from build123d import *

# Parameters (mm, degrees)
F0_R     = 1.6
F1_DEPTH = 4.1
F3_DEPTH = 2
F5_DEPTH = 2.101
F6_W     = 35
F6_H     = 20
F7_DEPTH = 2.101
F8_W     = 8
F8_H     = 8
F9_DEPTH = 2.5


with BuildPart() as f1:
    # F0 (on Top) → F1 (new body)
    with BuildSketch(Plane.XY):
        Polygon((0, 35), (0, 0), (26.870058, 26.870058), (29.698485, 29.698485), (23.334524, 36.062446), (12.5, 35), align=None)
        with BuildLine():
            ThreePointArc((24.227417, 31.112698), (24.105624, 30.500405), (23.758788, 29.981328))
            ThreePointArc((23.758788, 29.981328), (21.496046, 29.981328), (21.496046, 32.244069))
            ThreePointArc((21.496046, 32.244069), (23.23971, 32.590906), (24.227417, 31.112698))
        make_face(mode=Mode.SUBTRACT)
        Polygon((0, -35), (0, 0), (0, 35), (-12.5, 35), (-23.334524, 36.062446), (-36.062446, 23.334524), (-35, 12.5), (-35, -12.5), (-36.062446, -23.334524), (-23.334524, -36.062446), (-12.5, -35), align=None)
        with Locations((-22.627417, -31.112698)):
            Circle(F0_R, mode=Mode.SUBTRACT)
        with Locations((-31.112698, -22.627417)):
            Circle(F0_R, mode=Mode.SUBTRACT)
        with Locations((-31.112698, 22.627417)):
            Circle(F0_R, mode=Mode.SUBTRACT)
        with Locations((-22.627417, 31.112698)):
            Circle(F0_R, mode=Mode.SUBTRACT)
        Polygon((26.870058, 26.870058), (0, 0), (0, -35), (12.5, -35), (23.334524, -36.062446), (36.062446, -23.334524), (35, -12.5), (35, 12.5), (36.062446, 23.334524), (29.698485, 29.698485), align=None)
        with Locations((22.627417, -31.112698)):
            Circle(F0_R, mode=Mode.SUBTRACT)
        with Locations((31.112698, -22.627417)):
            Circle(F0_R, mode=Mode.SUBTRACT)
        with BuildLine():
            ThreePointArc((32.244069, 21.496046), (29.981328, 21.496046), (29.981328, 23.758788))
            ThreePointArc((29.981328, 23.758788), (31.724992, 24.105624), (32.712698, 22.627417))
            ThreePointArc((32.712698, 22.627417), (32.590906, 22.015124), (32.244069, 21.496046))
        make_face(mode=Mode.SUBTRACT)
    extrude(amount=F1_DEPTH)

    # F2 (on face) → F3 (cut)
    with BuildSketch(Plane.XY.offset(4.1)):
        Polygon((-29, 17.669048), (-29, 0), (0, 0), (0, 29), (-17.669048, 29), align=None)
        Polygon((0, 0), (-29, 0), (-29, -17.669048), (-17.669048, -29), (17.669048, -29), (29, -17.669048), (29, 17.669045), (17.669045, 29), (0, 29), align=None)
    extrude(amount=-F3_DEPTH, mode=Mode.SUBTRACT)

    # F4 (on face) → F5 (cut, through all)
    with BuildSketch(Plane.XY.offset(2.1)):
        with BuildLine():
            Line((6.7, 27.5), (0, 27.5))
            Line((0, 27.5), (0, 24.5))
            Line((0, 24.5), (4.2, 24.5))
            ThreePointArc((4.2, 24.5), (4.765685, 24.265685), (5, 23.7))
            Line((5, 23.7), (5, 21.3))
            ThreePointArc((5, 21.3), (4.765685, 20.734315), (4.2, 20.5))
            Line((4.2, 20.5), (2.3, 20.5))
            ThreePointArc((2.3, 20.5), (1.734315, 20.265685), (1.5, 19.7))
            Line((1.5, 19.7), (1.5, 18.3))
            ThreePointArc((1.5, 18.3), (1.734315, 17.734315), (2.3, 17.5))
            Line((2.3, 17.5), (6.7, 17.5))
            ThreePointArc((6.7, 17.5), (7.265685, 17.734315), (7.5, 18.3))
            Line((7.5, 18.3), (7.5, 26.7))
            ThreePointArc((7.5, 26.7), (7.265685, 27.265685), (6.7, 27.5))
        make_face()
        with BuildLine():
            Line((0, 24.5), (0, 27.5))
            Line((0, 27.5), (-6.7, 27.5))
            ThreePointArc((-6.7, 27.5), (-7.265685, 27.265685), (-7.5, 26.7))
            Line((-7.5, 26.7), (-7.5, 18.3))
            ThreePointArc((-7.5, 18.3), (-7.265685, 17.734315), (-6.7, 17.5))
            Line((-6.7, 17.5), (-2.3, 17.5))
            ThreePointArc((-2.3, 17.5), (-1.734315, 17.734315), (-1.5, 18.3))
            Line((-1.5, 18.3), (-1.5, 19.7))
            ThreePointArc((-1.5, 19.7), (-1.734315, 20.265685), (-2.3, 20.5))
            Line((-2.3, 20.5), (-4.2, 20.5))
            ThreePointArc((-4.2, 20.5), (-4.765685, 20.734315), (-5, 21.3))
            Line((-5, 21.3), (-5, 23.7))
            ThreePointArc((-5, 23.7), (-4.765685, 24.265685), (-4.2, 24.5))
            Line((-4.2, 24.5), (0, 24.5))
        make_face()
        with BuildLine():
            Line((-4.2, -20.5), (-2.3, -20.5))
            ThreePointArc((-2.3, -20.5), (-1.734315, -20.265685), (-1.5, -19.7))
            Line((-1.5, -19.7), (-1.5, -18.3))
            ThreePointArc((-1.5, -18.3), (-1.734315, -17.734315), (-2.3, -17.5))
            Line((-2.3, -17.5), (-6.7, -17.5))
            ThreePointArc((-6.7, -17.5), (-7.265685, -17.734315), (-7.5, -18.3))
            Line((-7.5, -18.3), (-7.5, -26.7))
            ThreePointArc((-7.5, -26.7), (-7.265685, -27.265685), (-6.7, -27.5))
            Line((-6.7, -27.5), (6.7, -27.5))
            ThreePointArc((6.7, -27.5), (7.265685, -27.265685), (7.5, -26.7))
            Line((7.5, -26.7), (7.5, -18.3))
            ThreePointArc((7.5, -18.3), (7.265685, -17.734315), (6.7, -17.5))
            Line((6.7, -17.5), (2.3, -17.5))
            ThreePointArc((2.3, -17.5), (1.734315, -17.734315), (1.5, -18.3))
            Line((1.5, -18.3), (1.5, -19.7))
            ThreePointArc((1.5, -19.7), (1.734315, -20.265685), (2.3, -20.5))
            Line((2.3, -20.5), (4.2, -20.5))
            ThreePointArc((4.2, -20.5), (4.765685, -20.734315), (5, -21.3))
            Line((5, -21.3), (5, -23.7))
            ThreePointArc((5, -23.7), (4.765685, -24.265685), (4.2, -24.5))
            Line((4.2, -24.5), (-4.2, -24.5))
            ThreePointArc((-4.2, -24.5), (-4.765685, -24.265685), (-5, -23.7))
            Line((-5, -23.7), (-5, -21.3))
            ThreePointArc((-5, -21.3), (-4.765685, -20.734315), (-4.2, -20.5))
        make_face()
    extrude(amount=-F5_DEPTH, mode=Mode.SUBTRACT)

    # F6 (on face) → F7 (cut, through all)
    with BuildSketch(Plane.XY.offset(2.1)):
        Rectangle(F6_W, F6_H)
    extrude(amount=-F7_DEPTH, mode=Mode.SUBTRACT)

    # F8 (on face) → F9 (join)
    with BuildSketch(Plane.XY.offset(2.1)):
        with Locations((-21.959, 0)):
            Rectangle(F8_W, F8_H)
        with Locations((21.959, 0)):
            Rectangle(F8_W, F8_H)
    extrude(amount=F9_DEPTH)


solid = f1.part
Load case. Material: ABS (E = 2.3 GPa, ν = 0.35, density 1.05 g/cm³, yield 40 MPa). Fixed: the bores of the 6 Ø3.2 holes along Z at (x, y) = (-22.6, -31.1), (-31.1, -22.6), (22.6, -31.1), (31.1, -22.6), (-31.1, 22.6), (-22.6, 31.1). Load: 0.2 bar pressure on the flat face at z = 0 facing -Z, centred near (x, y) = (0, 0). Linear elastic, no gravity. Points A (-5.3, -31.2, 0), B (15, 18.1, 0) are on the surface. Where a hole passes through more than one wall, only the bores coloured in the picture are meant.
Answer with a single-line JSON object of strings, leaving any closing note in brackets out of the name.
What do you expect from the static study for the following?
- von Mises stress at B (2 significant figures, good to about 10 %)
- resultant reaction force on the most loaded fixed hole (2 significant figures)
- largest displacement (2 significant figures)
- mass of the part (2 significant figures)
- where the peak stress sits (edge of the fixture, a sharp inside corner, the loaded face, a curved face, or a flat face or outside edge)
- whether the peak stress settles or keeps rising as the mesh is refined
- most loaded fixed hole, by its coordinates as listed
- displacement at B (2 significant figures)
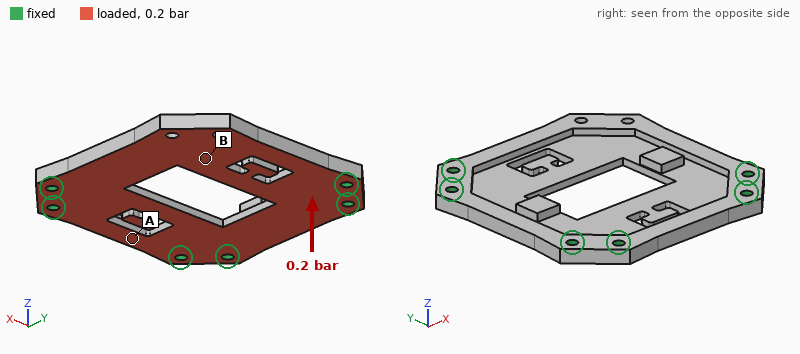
{"von Mises stress at B": "3.3 MPa", "resultant reaction force on the most loaded fixed hole": "40 N", "largest displacement": "1.1 mm", "mass of the part": "12 g", "where the peak stress sits": "edge of the fixture", "whether the peak stress settles or keeps rising as the mesh is refined": "keeps rising", "most loaded fixed hole, by its coordinates as listed": "(31.1, -22.6)", "displacement at B": "0.68 mm"}
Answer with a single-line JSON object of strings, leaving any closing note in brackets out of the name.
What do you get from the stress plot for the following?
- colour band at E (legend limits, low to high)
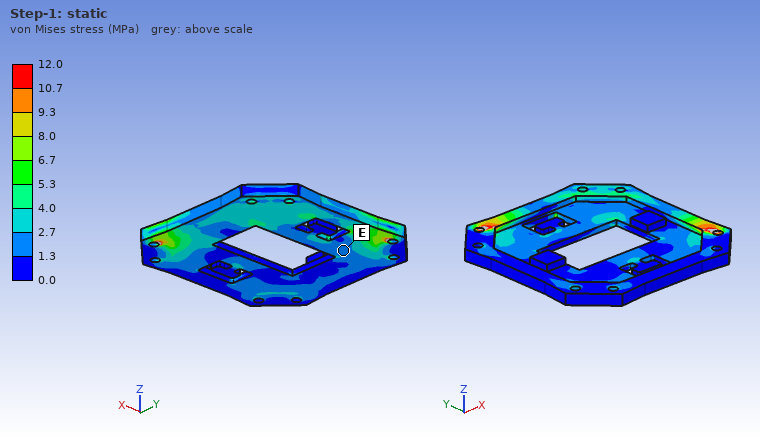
{"colour band at E": "1.3 to 2.7 MPa"}
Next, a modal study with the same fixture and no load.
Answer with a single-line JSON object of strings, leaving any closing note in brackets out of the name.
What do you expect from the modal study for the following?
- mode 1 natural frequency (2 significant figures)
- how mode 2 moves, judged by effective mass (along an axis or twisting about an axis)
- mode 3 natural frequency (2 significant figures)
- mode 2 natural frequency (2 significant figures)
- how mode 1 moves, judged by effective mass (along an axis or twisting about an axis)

{"mode 1 natural frequency": "460 Hz", "how mode 2 moves, judged by effective mass": "along Z", "mode 3 natural frequency": "1500 Hz", "mode 2 natural frequency": "1300 Hz", "how mode 1 moves, judged by effective mass": "along Z"}
